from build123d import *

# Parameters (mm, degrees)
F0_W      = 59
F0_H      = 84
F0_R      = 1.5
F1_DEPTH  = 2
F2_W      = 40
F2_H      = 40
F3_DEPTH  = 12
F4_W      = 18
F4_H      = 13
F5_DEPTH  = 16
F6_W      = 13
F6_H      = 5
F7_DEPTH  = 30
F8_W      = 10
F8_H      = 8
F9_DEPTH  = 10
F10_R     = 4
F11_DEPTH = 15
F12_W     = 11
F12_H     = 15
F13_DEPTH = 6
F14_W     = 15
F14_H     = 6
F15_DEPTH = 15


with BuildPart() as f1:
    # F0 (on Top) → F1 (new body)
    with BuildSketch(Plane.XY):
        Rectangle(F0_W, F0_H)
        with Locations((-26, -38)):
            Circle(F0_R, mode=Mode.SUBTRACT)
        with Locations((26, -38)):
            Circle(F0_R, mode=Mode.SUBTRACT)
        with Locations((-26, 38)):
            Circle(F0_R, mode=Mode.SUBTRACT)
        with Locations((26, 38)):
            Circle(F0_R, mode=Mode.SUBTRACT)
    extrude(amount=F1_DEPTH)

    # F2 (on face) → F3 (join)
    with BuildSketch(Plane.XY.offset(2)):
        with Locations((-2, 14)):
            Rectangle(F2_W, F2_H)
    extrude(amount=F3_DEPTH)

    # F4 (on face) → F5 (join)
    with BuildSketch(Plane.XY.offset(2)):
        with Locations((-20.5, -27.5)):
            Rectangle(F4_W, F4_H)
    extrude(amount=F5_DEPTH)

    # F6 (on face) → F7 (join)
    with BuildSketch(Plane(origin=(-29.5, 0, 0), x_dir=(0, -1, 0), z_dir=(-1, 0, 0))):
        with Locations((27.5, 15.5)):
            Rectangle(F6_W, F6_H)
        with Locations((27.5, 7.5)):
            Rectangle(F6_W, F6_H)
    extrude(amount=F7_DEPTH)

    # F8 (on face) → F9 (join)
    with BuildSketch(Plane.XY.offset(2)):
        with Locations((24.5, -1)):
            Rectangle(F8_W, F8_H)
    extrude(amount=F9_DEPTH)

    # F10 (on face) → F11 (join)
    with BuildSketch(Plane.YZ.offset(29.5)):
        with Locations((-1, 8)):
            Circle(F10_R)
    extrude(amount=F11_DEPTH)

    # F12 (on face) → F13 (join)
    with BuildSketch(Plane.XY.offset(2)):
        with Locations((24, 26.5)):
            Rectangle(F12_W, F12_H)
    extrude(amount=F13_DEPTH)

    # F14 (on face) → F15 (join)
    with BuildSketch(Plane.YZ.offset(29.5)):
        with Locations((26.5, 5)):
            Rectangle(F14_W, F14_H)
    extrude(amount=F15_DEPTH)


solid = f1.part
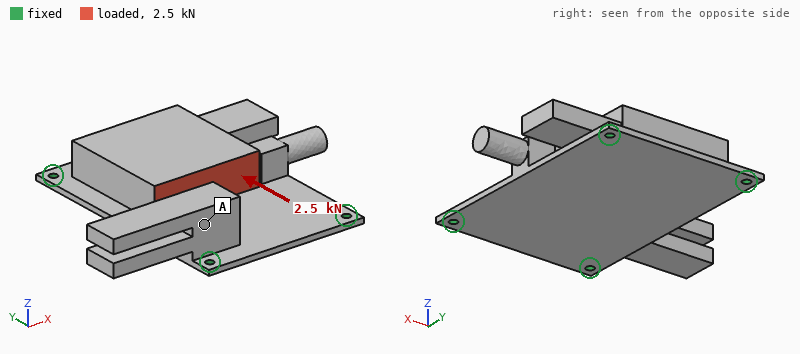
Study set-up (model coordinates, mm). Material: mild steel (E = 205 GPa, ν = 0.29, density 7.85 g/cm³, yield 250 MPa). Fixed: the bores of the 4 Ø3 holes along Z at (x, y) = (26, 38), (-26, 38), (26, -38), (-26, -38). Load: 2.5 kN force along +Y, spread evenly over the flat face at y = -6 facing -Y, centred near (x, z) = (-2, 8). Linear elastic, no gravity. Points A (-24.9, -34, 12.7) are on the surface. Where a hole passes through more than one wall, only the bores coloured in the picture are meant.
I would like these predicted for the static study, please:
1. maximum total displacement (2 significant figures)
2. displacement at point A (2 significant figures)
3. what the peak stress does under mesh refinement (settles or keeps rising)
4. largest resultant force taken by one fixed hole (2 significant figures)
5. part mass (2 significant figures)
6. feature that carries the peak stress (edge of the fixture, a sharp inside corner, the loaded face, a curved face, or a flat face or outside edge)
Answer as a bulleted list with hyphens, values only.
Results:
- 96 µm
- 45 µm
- keeps rising
- 810 N
- 320 g
- edge of the fixture
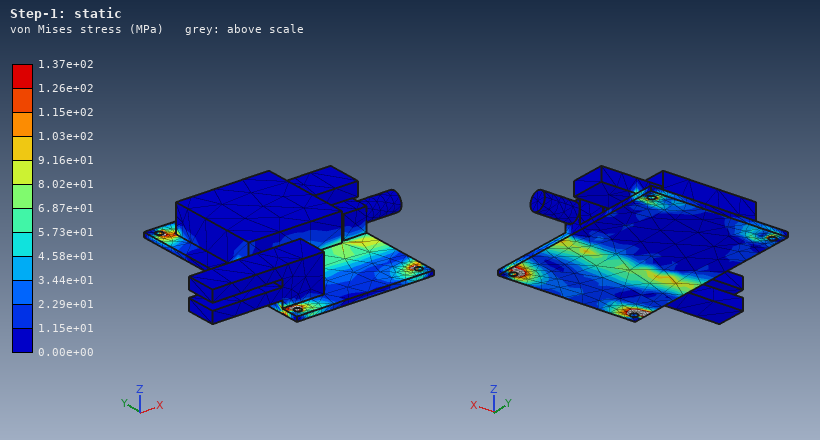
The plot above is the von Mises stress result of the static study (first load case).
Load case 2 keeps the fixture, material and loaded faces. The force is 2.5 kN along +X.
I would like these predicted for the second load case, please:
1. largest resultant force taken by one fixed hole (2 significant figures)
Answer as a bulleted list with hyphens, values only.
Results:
- 1.1 kN
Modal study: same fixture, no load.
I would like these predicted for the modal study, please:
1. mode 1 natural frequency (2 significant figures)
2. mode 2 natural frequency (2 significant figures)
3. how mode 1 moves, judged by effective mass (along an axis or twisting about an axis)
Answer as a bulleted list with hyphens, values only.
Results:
- 980 Hz
- 1400 Hz
- along Z
